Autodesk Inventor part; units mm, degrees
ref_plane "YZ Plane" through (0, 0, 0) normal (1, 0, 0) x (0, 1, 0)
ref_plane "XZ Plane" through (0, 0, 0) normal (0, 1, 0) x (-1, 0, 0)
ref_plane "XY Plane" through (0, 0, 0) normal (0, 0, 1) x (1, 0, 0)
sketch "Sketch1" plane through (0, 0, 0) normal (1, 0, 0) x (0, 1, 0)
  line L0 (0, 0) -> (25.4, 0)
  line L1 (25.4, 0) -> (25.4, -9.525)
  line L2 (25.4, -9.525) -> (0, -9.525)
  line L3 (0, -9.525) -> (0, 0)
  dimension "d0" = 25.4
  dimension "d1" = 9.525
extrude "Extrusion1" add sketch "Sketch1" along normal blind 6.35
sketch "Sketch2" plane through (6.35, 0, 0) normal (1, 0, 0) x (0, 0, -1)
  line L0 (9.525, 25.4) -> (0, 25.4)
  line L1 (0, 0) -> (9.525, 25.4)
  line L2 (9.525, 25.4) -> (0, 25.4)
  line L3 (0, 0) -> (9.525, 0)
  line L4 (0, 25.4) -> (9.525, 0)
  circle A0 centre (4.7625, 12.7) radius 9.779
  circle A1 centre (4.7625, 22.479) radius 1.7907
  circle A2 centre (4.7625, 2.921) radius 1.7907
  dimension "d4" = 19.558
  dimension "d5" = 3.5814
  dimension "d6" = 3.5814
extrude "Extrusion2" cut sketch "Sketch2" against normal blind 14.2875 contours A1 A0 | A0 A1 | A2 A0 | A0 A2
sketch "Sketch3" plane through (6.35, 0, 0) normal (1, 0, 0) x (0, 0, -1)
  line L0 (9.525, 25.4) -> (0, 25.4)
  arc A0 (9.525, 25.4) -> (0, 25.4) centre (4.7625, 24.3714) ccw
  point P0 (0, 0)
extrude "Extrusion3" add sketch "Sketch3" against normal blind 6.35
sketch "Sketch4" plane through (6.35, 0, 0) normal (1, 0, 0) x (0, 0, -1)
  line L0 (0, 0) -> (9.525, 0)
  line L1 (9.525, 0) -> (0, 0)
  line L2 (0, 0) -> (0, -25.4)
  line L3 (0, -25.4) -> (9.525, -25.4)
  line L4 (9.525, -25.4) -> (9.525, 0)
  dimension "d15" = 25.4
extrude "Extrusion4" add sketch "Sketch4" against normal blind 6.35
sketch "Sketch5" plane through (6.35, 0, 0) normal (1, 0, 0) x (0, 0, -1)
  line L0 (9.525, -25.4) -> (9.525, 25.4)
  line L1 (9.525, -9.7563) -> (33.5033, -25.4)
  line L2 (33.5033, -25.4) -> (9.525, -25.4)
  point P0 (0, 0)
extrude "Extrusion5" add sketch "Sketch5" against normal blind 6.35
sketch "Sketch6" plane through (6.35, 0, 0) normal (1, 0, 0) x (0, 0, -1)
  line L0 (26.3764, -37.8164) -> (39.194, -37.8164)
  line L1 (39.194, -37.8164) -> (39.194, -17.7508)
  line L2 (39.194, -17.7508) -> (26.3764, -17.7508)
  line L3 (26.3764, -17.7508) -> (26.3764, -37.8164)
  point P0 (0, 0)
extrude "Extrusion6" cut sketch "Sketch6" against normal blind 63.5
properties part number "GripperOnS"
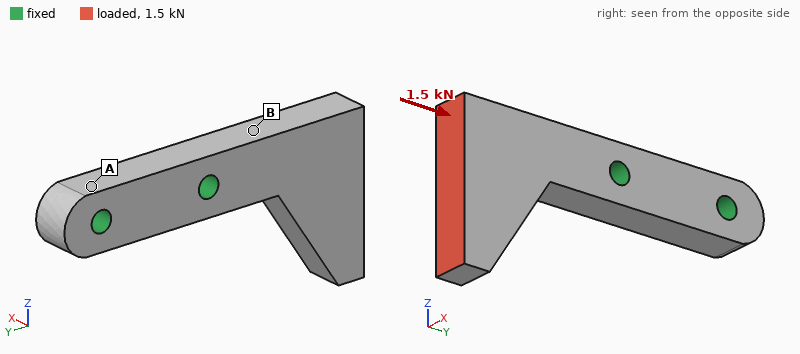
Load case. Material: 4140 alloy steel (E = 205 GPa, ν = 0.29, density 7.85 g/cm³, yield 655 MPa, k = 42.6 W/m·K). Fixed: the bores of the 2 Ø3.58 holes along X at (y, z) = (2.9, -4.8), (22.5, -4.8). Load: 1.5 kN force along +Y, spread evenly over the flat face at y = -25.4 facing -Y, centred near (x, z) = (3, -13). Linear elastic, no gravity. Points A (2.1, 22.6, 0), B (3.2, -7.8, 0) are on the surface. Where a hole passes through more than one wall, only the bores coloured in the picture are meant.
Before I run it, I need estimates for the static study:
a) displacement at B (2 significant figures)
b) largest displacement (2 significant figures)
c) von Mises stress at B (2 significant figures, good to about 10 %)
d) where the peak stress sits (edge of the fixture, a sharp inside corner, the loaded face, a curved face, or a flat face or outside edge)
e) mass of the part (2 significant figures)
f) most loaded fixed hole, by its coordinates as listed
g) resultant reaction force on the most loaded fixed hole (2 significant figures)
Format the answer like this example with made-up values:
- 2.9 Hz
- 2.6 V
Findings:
- 13 µm
- 84 µm
- 100 MPa
- edge of the fixture
- 33 g
- (2.9, -4.8)
- 1.5 kN
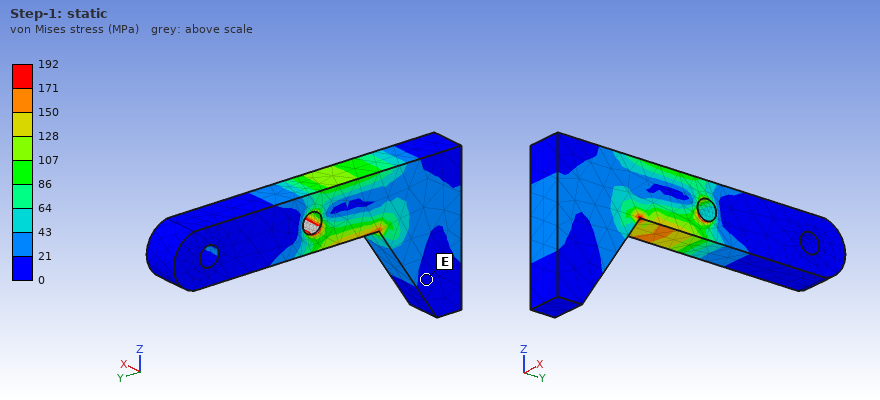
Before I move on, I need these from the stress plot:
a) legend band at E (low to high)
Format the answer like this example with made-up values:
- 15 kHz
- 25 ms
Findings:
- 0 to 21 MPa
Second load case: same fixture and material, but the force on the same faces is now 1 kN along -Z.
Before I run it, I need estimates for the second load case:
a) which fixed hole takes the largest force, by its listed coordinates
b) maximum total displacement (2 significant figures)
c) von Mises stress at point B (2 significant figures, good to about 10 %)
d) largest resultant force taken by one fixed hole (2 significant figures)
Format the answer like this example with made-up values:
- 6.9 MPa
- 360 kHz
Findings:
- (2.9, -4.8)
- 0.14 mm
- 180 MPa
- 1.5 kN
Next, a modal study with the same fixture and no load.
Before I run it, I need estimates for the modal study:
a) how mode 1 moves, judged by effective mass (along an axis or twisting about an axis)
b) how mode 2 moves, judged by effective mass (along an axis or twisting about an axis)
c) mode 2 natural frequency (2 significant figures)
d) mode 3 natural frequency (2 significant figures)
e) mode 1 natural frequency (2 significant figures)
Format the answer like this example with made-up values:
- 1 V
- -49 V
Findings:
- along X
- along Z
- 4700 Hz
- 9200 Hz
- 3800 Hz
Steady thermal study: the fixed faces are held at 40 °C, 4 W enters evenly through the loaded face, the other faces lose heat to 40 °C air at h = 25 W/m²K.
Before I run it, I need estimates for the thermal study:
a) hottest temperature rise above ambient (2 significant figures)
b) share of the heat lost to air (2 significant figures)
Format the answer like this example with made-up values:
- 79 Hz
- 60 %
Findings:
- 34 K
- 16 %
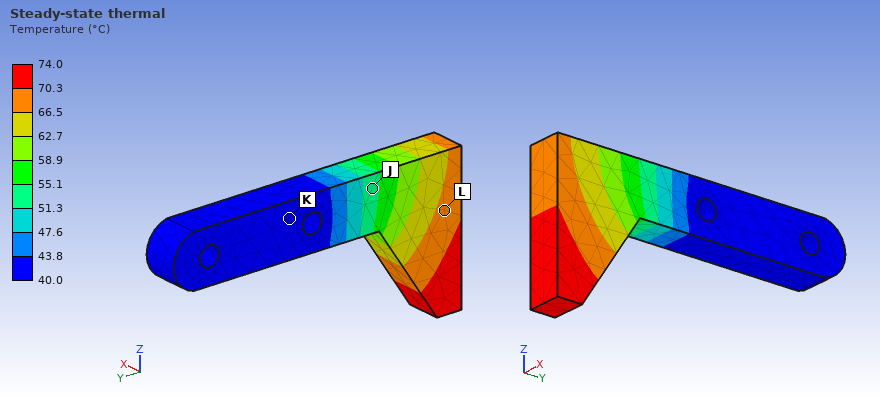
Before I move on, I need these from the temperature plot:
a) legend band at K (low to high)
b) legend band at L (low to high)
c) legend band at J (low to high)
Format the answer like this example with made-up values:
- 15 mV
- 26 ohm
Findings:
- 40.0 to 43.8 °C
- 66.5 to 70.3 °C
- 51.3 to 55.1 °C
